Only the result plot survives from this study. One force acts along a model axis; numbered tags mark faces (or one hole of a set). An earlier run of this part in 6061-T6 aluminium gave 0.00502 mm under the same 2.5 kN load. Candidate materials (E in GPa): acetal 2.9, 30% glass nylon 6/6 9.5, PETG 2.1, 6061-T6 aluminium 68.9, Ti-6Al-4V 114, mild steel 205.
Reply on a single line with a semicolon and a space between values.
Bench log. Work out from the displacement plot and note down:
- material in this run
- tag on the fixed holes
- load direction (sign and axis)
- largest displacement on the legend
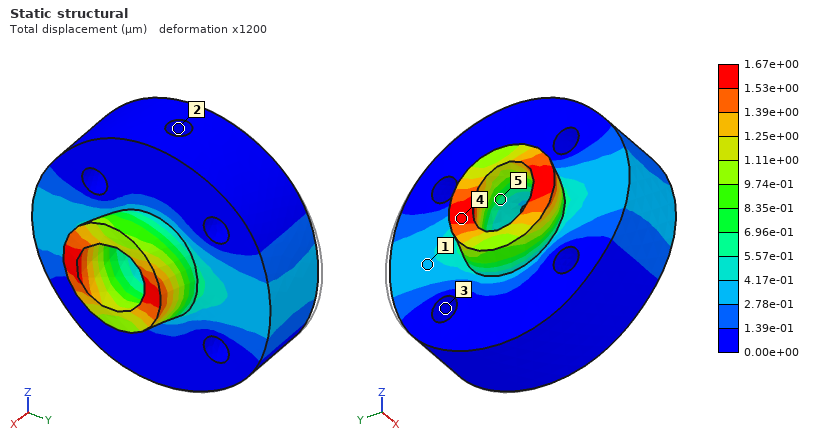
mild steel; 3; -Y; 1.67e+00 µm
